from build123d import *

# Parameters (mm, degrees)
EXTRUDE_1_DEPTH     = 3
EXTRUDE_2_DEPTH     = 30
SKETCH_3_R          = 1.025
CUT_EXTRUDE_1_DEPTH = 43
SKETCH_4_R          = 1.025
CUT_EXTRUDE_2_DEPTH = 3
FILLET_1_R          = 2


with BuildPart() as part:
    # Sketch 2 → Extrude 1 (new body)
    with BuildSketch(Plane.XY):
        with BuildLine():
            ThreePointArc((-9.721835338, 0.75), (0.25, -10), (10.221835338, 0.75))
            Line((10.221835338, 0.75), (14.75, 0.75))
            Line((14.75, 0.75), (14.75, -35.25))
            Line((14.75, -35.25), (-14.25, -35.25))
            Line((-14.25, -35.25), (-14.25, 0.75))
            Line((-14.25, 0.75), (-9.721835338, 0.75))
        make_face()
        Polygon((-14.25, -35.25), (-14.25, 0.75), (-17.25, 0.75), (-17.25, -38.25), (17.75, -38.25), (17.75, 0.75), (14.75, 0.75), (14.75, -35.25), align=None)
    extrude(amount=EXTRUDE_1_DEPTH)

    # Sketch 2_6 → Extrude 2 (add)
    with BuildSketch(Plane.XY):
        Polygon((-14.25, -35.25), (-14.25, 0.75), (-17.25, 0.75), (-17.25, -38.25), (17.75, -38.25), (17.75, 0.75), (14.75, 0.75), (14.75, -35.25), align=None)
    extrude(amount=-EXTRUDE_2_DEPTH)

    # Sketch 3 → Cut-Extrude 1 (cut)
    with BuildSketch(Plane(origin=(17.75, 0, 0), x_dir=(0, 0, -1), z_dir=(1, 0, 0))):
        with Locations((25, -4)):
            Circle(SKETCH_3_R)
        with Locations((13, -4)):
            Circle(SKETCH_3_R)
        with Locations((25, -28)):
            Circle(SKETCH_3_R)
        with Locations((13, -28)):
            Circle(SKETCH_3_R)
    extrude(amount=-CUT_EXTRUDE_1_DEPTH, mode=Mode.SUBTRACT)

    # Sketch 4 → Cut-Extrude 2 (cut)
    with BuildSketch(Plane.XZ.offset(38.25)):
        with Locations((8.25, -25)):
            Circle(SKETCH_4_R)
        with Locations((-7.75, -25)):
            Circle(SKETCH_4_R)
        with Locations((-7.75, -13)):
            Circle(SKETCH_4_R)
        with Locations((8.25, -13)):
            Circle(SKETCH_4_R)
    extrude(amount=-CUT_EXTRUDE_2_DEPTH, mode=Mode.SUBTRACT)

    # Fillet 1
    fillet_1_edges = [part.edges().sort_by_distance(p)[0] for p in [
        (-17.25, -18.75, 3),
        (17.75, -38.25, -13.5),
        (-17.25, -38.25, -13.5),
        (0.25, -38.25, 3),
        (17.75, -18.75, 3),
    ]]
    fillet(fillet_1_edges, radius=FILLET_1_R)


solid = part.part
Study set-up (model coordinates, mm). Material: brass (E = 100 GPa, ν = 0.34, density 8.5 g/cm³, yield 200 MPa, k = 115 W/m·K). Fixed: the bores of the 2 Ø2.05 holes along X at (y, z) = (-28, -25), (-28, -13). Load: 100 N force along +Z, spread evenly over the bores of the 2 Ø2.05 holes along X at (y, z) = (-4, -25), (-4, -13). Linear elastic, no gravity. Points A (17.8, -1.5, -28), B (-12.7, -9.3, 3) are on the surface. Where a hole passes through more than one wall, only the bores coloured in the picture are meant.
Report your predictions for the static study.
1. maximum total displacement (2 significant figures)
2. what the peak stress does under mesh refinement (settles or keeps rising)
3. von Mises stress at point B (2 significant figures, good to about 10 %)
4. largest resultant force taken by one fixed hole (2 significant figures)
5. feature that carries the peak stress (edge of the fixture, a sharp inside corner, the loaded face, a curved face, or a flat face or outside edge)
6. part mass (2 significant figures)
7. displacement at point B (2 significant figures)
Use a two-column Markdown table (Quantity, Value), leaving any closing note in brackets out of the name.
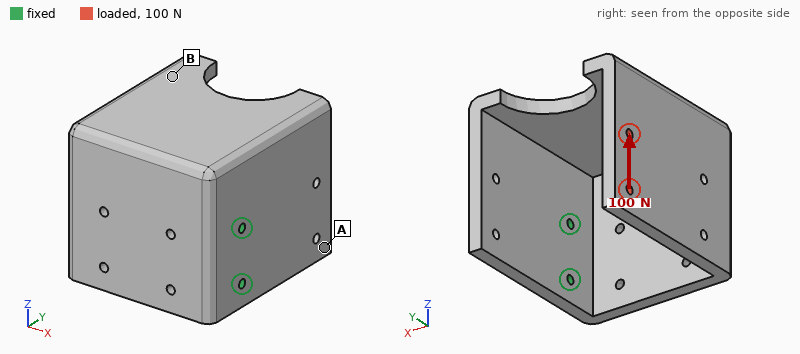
| Quantity | Value |
|---|---|
| maximum total displacement | 0.15 mm |
| what the peak stress does under mesh refinement | keeps rising |
| von Mises stress at point B | 17 MPa |
| largest resultant force taken by one fixed hole | 280 N |
| feature that carries the peak stress | edge of the fixture |
| part mass | 110 g |
| displacement at point B | 0.10 mm |
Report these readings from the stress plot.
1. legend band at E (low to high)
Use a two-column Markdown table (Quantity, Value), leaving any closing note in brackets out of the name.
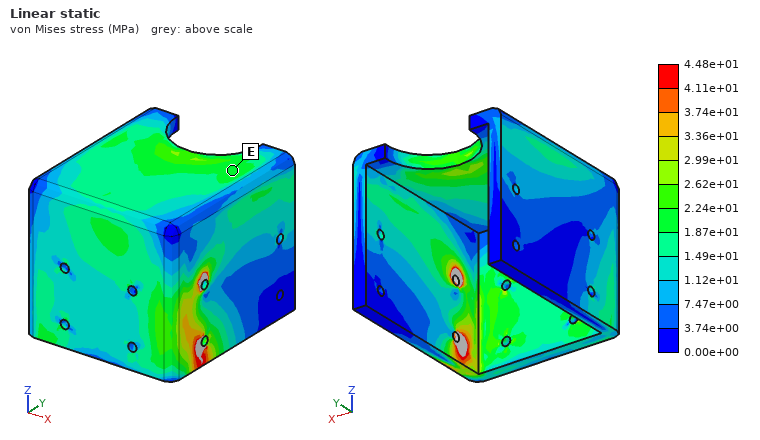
| Quantity | Value |
|---|---|
| legend band at E | 1.87e+01 to 2.24e+01 MPa |
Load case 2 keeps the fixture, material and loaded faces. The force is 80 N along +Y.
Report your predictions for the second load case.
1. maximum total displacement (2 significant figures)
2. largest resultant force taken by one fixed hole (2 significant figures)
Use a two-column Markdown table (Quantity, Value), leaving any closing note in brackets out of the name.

| Quantity | Value |
|---|---|
| maximum total displacement | 0.16 mm |
| largest resultant force taken by one fixed hole | 40 N |
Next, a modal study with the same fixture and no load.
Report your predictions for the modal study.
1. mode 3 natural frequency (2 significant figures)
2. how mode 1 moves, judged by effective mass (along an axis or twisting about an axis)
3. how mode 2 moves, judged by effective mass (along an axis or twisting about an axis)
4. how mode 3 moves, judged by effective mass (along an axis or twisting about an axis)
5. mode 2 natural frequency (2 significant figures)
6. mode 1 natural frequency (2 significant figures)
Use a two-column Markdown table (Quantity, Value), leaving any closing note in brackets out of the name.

| Quantity | Value |
|---|---|
| mode 3 natural frequency | 1800 Hz |
| how mode 1 moves, judged by effective mass | along Y |
| how mode 2 moves, judged by effective mass | along Z |
| how mode 3 moves, judged by effective mass | along X |
| mode 2 natural frequency | 890 Hz |
| mode 1 natural frequency | 600 Hz |
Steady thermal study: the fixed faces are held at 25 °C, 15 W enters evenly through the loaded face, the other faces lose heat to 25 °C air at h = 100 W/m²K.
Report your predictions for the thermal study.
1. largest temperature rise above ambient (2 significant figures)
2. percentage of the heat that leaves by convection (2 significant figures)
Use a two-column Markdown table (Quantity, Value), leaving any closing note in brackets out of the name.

| Quantity | Value |
|---|---|
| largest temperature rise above ambient | 46 K |
| percentage of the heat that leaves by convection | 71 % |
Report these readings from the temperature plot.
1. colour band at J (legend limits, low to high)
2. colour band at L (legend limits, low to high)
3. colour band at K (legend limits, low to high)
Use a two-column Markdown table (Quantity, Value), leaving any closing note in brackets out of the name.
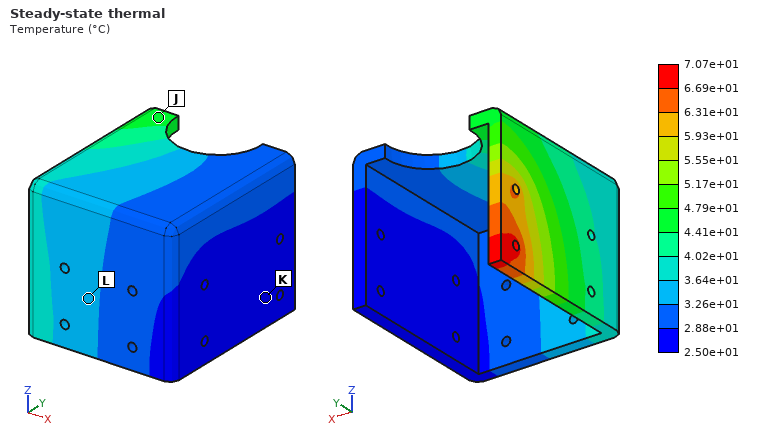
| Quantity | Value |
|---|---|
| colour band at J | 4.41e+01 to 4.79e+01 °C |
| colour band at L | 3.26e+01 to 3.64e+01 °C |
| colour band at K | 2.50e+01 to 2.88e+01 °C |
